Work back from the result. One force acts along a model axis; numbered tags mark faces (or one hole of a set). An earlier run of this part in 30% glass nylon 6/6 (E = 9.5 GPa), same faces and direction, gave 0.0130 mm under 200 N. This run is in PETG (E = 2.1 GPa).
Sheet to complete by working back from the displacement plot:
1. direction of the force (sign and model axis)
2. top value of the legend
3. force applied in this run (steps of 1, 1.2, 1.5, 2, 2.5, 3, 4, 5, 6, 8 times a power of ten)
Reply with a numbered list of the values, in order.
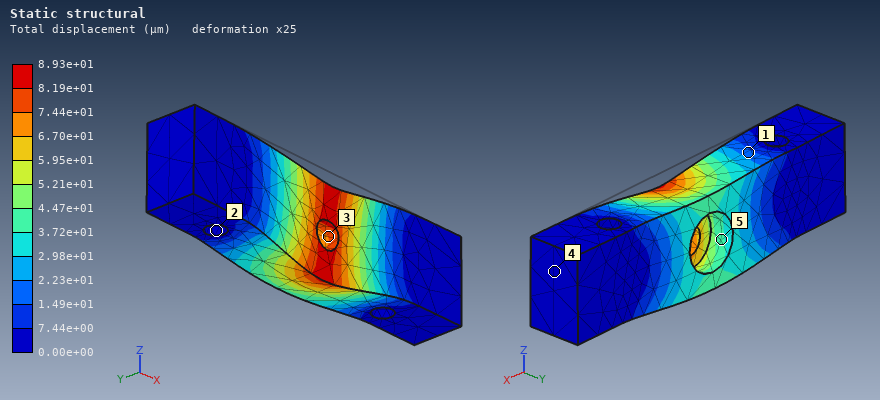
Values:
1. -Z
2. 8.93e+01 µm
3. 300 N
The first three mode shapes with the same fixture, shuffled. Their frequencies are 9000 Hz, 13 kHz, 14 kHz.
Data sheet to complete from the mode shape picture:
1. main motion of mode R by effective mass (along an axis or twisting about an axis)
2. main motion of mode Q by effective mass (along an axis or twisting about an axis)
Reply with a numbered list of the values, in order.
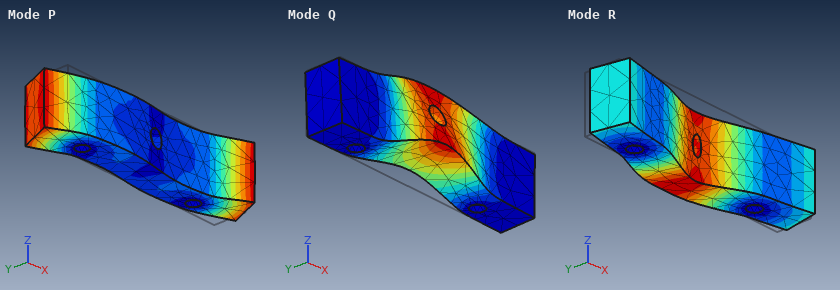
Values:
1. along Y
2. along Z
